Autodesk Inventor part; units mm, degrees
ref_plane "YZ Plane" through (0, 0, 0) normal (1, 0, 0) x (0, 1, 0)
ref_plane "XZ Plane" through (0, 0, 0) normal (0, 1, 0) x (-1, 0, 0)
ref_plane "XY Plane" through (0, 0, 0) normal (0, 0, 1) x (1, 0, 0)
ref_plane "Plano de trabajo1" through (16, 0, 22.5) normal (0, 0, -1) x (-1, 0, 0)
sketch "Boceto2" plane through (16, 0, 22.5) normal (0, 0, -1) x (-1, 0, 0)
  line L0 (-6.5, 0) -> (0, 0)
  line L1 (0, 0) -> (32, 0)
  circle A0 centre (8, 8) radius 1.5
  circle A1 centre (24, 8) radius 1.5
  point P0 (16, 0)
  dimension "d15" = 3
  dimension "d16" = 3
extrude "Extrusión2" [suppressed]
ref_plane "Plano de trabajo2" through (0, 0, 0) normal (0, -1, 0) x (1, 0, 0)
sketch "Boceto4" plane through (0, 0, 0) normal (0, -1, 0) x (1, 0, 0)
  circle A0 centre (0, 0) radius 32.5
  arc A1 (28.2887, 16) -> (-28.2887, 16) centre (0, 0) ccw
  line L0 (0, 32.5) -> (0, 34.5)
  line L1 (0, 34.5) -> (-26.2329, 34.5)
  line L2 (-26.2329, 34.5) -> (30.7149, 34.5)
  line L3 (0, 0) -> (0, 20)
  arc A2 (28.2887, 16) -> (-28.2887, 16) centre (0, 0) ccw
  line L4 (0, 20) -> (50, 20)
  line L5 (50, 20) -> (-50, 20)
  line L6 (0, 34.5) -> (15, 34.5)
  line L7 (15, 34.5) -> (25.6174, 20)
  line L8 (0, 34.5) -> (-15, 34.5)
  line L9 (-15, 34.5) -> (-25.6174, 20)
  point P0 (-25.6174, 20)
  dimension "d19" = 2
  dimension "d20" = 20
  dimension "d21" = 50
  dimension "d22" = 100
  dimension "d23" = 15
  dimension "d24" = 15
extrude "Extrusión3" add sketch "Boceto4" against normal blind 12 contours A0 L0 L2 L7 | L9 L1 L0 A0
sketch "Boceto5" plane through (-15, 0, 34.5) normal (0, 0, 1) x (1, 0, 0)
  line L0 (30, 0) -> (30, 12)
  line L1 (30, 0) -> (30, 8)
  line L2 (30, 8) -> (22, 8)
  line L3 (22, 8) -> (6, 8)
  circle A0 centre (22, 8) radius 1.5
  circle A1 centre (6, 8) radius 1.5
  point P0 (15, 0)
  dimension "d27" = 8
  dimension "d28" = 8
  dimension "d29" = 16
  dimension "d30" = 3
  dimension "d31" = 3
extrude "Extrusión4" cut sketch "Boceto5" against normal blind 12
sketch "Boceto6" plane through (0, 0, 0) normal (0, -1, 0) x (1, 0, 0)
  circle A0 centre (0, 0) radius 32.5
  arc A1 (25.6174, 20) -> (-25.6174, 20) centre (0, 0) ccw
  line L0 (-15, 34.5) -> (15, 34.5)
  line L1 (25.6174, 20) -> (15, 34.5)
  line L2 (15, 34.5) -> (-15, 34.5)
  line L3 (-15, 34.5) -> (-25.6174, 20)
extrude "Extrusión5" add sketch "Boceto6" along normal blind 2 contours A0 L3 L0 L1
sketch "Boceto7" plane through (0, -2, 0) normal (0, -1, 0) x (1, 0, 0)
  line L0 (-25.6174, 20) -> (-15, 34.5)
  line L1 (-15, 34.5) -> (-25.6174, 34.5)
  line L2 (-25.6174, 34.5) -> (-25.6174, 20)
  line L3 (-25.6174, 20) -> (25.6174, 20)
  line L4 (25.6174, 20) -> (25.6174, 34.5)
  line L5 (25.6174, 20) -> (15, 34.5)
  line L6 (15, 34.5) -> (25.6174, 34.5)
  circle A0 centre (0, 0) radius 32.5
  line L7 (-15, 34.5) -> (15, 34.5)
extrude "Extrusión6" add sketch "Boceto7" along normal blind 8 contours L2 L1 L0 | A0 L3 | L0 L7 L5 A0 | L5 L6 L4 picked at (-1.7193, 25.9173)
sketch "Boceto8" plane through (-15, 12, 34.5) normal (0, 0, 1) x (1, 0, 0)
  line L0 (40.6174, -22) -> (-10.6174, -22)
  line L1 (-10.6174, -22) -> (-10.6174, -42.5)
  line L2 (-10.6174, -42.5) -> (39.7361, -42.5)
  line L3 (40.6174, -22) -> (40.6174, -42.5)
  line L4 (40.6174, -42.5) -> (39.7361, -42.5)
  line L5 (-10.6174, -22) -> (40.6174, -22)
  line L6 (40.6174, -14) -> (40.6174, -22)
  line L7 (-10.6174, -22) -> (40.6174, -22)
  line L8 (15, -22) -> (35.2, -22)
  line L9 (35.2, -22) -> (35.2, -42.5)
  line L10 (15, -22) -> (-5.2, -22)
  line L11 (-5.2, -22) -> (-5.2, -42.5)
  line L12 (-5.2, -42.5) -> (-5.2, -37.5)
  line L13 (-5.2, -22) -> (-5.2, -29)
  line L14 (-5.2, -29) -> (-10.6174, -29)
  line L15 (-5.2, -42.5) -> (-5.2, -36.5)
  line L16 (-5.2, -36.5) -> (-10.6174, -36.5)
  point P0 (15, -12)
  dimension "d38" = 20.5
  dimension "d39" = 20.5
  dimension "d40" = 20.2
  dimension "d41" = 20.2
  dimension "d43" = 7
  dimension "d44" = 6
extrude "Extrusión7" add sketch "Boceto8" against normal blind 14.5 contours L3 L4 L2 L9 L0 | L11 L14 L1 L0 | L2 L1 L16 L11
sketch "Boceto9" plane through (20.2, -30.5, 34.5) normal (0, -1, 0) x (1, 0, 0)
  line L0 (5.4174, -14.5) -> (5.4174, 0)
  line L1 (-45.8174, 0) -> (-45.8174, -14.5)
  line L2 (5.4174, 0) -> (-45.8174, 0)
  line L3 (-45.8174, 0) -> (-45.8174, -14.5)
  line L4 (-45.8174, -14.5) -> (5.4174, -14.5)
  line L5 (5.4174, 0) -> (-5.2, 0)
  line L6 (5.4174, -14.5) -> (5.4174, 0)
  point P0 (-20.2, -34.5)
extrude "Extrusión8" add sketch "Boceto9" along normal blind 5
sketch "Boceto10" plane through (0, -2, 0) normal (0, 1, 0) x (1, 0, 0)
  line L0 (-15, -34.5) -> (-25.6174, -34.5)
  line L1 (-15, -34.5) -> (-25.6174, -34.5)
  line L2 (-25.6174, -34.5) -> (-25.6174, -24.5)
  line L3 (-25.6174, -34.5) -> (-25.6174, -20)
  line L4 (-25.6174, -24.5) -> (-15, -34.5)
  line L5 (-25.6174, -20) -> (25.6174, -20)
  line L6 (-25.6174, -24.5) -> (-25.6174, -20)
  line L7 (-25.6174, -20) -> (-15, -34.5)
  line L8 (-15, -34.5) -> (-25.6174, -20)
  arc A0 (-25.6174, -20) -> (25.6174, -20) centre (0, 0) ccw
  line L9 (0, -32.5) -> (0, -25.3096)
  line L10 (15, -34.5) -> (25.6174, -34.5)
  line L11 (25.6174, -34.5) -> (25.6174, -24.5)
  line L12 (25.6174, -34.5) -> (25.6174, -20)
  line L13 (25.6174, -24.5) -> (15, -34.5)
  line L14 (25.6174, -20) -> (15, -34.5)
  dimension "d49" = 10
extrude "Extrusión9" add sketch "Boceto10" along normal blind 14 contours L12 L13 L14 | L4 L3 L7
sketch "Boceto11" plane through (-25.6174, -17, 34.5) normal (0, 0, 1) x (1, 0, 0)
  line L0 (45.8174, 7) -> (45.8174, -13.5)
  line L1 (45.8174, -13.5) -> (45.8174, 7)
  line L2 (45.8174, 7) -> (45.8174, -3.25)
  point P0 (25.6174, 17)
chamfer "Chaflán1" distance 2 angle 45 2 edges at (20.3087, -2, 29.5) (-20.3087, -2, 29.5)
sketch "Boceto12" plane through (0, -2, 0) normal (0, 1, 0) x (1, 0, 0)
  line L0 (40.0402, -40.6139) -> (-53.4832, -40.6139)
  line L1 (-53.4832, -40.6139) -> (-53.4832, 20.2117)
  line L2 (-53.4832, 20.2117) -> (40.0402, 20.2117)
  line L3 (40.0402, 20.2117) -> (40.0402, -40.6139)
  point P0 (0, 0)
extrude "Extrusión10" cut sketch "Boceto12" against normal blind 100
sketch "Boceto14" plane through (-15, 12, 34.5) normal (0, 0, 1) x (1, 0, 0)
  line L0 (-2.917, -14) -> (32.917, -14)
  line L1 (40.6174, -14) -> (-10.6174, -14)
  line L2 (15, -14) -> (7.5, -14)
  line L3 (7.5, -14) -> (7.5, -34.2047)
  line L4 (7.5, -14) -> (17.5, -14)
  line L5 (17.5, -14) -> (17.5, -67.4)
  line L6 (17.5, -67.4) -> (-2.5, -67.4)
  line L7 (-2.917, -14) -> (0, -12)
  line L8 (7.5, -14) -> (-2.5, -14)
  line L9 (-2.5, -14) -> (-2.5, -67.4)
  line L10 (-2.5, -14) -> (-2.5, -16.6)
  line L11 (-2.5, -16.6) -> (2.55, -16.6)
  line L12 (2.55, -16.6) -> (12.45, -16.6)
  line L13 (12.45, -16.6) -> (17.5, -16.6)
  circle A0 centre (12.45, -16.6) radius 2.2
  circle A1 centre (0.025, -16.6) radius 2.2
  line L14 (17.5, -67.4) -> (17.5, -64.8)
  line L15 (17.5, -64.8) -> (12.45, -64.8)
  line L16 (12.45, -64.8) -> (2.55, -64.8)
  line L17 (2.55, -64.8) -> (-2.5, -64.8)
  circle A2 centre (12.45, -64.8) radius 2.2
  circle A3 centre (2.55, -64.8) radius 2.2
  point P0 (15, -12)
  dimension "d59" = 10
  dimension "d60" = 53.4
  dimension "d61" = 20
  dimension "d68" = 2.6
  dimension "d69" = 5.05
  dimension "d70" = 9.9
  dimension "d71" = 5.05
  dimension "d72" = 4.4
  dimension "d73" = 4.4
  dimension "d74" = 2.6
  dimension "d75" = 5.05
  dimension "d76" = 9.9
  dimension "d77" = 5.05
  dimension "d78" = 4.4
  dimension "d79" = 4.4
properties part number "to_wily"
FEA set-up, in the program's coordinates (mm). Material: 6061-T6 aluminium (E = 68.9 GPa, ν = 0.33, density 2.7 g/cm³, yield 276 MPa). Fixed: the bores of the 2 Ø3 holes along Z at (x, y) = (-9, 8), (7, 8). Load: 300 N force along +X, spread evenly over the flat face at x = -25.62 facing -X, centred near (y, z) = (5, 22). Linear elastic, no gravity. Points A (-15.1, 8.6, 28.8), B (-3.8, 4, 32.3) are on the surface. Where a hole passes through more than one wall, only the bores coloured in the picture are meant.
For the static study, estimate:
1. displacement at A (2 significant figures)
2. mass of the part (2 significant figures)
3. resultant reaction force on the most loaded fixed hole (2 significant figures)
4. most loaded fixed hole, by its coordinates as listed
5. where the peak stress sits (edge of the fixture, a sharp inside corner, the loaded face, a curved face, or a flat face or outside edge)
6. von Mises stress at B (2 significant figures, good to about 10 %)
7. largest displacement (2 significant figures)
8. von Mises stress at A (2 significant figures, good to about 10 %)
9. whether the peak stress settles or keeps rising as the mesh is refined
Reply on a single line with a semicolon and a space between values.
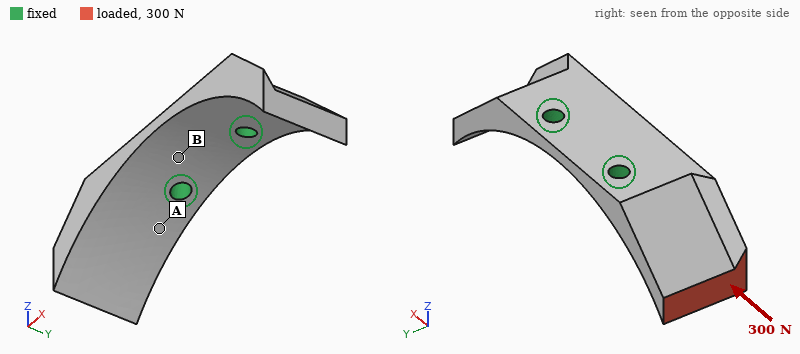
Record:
0.020 mm; 7.2 g; 290 N; (-9, 8); edge of the fixture; 18 MPa; 0.13 mm; 69 MPa; keeps rising
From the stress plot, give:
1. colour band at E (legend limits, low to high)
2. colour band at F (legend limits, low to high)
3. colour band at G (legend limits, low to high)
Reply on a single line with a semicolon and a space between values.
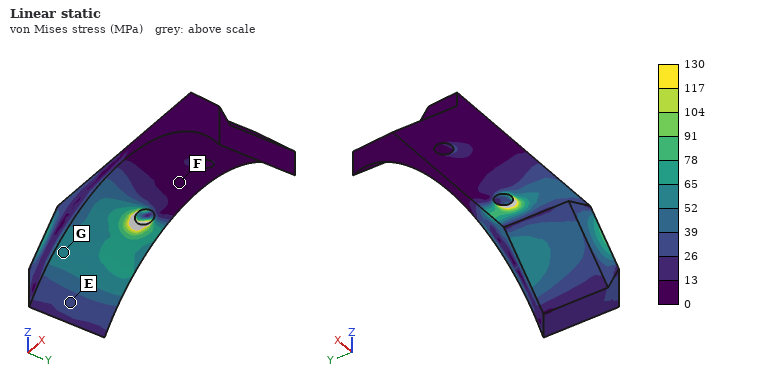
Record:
26 to 39 MPa; 0 to 13 MPa; 52 to 65 MPa
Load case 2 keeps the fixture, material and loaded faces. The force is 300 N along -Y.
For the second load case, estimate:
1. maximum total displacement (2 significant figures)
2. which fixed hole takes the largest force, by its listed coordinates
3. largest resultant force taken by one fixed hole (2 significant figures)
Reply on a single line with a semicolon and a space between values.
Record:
68 µm; (-9, 8); 520 N
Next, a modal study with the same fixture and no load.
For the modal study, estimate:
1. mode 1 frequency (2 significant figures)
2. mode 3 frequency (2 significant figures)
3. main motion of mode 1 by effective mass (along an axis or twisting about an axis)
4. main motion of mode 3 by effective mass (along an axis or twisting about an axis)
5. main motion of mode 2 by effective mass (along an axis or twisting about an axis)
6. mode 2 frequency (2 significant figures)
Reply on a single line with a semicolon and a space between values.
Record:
5700 Hz; 10 kHz; along Z; along Y; along Z; 8100 Hz
